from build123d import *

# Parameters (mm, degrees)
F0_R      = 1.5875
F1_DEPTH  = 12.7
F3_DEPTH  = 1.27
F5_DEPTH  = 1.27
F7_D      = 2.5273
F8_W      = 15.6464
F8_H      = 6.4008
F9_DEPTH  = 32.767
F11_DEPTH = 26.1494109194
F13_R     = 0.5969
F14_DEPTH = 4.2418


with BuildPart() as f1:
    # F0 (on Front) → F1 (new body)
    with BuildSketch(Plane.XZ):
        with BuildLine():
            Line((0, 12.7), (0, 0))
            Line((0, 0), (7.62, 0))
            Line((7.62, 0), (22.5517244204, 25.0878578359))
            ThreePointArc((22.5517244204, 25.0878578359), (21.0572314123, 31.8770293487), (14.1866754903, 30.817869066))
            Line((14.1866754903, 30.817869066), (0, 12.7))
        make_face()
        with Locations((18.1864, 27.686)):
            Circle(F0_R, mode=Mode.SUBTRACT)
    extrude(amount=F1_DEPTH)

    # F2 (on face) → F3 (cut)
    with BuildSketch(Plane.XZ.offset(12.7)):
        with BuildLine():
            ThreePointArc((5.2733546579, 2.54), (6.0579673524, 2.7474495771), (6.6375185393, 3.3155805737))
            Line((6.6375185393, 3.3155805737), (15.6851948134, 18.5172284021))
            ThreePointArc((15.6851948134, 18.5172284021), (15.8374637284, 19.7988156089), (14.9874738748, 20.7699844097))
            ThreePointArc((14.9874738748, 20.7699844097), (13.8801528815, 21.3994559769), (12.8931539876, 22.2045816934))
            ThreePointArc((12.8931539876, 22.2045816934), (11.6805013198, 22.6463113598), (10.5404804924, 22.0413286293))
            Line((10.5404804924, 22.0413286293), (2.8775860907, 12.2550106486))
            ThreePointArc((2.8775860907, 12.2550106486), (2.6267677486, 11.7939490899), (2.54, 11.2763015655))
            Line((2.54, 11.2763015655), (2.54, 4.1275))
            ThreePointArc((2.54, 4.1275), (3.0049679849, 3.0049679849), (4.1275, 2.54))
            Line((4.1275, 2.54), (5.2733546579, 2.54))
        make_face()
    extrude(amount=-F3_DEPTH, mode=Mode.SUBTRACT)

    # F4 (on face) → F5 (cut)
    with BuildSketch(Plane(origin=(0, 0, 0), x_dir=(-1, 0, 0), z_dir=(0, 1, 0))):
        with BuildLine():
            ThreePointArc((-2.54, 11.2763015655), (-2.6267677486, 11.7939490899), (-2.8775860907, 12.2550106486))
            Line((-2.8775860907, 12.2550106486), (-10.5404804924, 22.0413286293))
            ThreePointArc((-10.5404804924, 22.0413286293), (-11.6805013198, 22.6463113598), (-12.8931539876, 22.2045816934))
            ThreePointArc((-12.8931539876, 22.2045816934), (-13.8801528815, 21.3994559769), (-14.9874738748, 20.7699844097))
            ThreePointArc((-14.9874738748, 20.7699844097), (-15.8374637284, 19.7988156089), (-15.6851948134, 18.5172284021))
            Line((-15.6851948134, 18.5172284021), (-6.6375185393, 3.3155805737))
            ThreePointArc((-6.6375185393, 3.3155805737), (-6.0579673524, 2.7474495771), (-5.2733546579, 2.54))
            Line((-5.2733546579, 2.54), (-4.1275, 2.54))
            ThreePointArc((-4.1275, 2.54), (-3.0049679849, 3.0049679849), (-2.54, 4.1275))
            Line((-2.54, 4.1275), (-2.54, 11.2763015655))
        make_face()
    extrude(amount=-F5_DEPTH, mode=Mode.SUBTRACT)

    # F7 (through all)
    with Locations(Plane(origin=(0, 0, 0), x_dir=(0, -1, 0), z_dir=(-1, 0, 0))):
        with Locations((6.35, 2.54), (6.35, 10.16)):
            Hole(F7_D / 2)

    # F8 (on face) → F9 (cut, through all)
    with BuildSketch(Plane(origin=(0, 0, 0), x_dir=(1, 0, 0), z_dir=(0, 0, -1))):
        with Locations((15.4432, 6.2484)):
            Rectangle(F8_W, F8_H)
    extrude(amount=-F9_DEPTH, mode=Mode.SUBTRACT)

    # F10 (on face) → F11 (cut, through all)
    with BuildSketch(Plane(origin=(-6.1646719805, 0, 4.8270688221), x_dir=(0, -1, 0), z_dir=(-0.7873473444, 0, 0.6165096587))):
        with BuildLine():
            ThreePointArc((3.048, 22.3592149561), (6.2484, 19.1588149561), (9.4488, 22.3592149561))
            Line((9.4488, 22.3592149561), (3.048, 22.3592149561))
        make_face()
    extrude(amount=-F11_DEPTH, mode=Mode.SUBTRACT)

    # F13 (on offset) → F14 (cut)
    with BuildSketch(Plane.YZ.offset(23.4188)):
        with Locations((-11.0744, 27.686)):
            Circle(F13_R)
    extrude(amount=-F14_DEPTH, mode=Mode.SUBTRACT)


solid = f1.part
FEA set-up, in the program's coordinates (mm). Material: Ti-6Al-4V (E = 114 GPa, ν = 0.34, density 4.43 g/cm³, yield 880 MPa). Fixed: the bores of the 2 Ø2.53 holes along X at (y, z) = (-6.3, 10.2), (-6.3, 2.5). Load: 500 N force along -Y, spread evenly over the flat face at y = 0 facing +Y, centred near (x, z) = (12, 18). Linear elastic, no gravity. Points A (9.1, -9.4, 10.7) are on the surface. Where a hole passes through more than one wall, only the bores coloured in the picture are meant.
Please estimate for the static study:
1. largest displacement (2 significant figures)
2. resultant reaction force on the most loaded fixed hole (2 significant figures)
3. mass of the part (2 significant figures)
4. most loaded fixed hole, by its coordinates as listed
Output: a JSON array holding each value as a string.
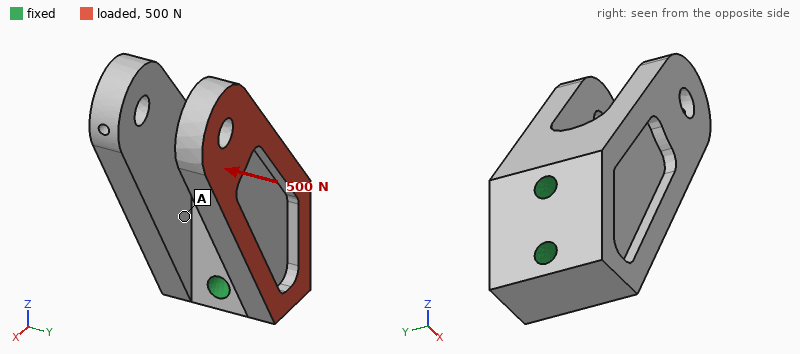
["0.26 mm", "790 N", "13 g", "(-6.3, 10.2)"]
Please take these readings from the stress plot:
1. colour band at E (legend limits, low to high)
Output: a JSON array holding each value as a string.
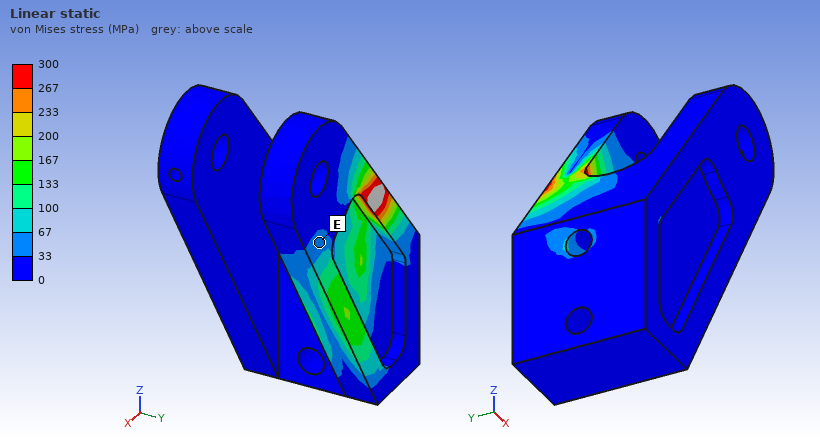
["33 to 67 MPa"]
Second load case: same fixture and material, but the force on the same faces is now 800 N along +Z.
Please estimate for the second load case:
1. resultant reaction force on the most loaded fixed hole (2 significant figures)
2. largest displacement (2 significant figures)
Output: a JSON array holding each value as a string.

["760 N", "58 µm"]
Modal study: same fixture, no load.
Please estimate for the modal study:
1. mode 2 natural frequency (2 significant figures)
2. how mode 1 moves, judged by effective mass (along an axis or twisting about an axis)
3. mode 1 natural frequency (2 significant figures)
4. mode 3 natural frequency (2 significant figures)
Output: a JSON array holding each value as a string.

["5200 Hz", "along Y", "4700 Hz", "12 kHz"]
